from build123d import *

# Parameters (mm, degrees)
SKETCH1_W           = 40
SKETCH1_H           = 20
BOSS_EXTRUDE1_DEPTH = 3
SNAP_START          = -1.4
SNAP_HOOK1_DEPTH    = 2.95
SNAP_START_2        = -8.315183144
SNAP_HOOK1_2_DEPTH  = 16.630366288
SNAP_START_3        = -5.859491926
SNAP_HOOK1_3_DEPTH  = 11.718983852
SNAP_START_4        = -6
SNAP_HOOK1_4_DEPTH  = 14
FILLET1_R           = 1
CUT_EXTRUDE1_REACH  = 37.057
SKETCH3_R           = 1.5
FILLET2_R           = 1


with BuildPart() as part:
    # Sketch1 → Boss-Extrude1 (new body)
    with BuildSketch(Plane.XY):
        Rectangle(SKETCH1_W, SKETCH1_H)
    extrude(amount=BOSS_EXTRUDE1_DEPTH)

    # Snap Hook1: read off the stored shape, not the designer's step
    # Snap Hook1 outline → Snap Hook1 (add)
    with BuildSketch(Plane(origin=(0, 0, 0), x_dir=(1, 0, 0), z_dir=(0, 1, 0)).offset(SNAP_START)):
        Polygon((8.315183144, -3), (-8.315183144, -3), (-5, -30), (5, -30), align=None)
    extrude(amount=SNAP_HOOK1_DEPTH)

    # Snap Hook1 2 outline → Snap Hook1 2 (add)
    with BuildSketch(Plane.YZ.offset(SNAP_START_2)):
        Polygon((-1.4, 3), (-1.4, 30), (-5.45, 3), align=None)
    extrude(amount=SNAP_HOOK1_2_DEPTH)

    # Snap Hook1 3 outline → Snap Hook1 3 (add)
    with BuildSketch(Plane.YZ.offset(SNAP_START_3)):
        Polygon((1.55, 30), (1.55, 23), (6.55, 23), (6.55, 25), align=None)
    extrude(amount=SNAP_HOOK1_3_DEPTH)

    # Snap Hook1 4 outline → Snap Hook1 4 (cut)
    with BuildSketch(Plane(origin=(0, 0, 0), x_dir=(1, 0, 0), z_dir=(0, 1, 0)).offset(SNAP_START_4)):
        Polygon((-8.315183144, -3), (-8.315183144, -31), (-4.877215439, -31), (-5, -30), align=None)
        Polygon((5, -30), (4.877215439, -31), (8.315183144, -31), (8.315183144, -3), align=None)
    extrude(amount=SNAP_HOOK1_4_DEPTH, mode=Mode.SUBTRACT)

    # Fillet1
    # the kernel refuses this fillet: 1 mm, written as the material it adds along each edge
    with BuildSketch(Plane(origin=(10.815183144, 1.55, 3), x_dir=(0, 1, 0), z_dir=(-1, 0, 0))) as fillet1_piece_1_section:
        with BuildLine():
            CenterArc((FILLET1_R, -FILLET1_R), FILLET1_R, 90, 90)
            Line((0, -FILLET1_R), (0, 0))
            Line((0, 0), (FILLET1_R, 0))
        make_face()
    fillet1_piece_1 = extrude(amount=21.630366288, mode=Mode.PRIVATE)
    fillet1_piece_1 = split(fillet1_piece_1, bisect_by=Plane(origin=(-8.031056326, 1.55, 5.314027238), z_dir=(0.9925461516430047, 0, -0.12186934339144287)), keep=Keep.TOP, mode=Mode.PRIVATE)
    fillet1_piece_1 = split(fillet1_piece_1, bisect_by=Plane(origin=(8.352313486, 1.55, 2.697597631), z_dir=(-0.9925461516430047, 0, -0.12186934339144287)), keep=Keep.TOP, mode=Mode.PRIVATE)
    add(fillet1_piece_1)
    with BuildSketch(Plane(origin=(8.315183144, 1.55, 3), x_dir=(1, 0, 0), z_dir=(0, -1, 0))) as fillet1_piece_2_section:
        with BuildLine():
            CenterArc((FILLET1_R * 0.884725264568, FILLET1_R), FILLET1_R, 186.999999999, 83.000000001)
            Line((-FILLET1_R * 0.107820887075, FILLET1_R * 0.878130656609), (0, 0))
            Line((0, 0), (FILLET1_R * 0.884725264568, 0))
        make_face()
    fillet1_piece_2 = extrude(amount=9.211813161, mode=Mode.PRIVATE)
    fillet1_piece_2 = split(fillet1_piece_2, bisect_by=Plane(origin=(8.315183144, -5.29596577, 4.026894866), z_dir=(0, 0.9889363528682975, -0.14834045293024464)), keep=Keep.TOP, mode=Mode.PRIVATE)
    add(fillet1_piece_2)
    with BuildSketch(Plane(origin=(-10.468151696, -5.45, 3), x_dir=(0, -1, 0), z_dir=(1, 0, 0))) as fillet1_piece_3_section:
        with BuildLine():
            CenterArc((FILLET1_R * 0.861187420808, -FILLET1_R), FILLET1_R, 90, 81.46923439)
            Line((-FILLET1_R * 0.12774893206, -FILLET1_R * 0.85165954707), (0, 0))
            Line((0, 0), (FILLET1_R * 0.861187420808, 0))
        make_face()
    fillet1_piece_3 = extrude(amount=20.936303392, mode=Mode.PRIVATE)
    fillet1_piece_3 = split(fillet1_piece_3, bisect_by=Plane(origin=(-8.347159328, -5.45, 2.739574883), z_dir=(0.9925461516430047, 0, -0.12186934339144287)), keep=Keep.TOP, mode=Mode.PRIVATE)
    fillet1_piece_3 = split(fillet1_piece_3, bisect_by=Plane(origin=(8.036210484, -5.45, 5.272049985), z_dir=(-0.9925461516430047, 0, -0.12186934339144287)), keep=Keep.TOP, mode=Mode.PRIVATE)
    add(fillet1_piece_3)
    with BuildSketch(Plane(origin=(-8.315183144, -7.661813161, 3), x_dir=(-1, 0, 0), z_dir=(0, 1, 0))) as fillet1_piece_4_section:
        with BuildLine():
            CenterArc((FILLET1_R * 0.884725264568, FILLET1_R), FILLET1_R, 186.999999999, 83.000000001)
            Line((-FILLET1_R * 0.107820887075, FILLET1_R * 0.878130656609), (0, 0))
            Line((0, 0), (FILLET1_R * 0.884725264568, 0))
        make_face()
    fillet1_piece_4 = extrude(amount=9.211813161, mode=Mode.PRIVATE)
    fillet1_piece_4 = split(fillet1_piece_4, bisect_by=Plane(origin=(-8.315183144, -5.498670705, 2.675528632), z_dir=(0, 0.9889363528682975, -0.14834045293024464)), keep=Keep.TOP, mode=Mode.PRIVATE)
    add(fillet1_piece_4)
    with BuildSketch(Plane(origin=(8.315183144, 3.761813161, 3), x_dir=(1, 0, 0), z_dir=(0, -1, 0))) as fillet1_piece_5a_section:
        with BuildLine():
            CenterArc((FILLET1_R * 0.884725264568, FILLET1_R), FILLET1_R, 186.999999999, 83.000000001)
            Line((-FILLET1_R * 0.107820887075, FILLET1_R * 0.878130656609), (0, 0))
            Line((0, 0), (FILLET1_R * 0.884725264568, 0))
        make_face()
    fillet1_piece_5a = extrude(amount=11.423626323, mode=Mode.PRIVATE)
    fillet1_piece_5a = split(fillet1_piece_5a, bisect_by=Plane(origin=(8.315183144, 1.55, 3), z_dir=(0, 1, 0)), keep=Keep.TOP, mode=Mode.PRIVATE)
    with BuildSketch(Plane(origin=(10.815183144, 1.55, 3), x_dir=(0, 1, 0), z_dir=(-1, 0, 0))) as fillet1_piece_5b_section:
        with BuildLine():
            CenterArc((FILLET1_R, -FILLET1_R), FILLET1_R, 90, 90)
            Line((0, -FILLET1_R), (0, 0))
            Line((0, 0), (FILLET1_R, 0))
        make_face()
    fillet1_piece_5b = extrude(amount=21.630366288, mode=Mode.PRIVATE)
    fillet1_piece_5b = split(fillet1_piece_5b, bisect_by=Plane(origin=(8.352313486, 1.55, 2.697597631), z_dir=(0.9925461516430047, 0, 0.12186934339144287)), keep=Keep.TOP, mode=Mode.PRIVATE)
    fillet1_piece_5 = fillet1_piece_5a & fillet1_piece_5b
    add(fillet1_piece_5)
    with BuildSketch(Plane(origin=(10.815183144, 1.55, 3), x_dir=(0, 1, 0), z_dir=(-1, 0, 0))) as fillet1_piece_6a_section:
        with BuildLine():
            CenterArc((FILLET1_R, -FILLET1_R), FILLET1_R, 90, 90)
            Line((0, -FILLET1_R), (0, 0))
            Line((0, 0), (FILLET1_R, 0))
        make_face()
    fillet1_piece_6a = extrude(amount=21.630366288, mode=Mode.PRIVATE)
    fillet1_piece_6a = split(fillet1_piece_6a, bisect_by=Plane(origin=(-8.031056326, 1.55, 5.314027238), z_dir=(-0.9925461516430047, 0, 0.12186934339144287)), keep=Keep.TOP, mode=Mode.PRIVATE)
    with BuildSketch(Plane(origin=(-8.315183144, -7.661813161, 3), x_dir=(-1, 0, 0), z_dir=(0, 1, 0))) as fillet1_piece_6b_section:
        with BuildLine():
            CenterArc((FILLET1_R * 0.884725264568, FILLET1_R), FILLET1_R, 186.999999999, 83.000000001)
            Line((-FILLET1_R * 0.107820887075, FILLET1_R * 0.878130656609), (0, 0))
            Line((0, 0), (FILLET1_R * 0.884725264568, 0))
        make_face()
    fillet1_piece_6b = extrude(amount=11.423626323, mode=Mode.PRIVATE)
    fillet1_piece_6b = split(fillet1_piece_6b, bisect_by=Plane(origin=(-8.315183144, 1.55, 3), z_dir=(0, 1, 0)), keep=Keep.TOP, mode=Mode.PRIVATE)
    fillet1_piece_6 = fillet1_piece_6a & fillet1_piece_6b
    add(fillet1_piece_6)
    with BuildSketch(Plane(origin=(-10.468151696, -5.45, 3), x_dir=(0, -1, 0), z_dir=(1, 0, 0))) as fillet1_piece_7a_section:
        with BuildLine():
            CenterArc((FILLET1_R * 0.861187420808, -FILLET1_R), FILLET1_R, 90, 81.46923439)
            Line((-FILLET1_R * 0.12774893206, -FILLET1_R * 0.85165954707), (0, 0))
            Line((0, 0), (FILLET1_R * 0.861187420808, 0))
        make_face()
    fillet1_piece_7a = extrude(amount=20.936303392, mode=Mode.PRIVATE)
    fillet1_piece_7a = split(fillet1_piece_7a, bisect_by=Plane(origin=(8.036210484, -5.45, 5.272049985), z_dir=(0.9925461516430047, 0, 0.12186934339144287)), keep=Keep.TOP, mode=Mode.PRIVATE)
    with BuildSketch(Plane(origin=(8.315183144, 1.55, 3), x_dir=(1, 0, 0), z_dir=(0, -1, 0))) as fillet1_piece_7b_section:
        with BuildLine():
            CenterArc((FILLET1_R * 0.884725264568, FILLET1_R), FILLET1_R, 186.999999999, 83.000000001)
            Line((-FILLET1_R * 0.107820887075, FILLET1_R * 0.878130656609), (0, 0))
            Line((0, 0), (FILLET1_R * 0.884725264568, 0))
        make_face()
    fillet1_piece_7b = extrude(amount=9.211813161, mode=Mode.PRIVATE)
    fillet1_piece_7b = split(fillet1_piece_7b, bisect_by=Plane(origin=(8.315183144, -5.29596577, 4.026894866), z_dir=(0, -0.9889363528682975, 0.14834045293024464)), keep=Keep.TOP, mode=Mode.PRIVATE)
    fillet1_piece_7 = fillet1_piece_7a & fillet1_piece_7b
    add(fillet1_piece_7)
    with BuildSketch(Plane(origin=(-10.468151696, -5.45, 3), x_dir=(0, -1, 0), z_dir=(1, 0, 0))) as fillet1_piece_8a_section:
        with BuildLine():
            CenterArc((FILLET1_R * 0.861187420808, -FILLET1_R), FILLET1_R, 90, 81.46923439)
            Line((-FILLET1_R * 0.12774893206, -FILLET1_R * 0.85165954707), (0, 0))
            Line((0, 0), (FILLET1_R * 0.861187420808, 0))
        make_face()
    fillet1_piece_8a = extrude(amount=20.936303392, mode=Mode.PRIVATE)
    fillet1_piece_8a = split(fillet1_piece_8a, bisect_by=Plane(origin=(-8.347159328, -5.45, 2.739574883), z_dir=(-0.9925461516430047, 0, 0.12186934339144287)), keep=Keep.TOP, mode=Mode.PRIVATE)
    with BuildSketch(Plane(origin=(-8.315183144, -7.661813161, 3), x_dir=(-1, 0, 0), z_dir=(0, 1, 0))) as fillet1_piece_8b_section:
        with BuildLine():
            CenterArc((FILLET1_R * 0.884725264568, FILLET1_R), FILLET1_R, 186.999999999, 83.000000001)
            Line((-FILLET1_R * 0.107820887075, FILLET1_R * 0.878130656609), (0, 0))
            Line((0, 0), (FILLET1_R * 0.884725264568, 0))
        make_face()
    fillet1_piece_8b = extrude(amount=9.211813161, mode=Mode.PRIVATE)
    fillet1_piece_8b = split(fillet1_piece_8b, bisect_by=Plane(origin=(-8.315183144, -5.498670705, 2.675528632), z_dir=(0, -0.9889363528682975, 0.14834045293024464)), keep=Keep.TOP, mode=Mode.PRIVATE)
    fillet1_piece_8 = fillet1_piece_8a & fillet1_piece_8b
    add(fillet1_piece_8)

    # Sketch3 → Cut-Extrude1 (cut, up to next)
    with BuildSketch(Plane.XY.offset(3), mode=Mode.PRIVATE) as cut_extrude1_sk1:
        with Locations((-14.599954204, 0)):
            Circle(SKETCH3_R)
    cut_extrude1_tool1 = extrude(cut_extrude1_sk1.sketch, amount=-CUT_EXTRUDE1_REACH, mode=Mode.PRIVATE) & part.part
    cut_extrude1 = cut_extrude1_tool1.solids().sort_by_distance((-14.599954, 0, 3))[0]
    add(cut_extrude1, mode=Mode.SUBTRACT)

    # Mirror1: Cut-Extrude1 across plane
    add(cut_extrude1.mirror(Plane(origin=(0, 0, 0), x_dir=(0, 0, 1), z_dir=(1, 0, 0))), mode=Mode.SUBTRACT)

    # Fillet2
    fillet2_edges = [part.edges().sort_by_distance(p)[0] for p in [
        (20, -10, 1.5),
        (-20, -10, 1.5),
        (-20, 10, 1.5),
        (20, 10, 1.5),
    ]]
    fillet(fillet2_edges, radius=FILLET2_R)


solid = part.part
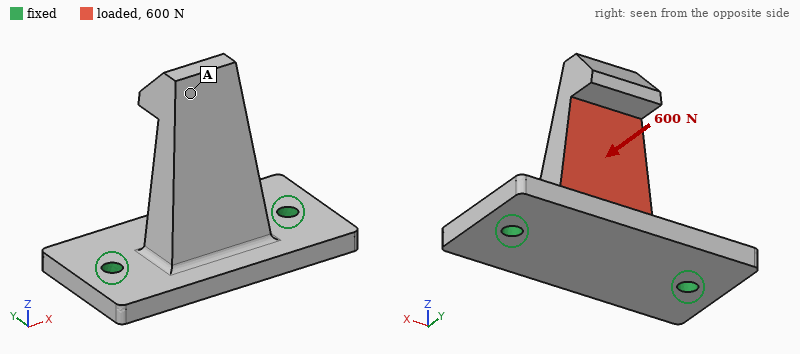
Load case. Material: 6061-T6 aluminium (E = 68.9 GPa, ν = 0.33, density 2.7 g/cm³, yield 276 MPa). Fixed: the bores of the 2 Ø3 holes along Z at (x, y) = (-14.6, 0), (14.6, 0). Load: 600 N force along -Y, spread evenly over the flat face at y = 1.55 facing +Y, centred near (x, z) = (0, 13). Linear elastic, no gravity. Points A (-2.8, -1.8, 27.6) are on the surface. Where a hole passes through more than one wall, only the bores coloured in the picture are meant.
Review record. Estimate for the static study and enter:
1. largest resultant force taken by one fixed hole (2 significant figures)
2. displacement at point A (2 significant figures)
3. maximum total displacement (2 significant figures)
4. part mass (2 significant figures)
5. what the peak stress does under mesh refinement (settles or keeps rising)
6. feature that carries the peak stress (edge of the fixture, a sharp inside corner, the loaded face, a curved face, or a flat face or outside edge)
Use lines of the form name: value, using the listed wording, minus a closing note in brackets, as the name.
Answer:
largest resultant force taken by one fixed hole: 300 N
displacement at point A: 0.21 mm
maximum total displacement: 0.23 mm
part mass: 12 g
what the peak stress does under mesh refinement: keeps rising
feature that carries the peak stress: edge of the fixture
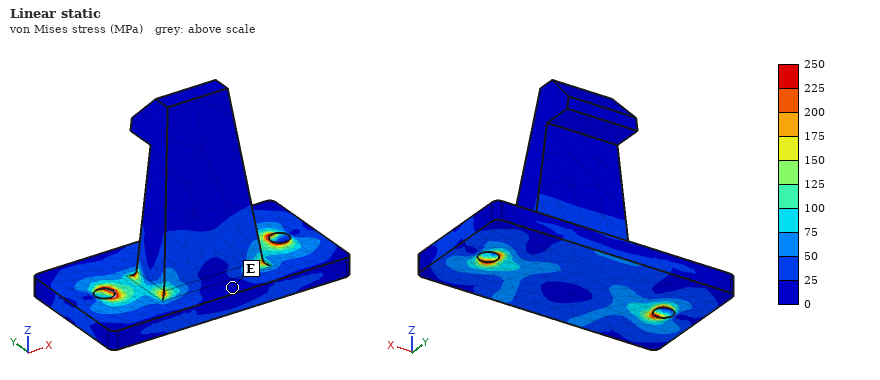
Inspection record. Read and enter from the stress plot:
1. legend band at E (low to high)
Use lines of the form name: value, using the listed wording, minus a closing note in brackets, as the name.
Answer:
legend band at E: 0 to 25 MPa
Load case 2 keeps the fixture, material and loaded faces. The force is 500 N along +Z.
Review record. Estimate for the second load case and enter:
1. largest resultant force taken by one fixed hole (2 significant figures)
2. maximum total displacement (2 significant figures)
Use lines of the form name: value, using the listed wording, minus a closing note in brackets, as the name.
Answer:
largest resultant force taken by one fixed hole: 270 N
maximum total displacement: 46 µm
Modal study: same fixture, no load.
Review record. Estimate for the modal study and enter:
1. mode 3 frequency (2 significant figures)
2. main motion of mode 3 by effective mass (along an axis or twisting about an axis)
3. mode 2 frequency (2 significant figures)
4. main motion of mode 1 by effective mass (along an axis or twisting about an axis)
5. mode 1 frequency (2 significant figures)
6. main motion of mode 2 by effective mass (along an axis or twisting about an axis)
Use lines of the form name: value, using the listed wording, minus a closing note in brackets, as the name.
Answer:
mode 3 frequency: 13 kHz
main motion of mode 3 by effective mass: along Z
mode 2 frequency: 9700 Hz
main motion of mode 1 by effective mass: along Y
mode 1 frequency: 3700 Hz
main motion of mode 2 by effective mass: along X
